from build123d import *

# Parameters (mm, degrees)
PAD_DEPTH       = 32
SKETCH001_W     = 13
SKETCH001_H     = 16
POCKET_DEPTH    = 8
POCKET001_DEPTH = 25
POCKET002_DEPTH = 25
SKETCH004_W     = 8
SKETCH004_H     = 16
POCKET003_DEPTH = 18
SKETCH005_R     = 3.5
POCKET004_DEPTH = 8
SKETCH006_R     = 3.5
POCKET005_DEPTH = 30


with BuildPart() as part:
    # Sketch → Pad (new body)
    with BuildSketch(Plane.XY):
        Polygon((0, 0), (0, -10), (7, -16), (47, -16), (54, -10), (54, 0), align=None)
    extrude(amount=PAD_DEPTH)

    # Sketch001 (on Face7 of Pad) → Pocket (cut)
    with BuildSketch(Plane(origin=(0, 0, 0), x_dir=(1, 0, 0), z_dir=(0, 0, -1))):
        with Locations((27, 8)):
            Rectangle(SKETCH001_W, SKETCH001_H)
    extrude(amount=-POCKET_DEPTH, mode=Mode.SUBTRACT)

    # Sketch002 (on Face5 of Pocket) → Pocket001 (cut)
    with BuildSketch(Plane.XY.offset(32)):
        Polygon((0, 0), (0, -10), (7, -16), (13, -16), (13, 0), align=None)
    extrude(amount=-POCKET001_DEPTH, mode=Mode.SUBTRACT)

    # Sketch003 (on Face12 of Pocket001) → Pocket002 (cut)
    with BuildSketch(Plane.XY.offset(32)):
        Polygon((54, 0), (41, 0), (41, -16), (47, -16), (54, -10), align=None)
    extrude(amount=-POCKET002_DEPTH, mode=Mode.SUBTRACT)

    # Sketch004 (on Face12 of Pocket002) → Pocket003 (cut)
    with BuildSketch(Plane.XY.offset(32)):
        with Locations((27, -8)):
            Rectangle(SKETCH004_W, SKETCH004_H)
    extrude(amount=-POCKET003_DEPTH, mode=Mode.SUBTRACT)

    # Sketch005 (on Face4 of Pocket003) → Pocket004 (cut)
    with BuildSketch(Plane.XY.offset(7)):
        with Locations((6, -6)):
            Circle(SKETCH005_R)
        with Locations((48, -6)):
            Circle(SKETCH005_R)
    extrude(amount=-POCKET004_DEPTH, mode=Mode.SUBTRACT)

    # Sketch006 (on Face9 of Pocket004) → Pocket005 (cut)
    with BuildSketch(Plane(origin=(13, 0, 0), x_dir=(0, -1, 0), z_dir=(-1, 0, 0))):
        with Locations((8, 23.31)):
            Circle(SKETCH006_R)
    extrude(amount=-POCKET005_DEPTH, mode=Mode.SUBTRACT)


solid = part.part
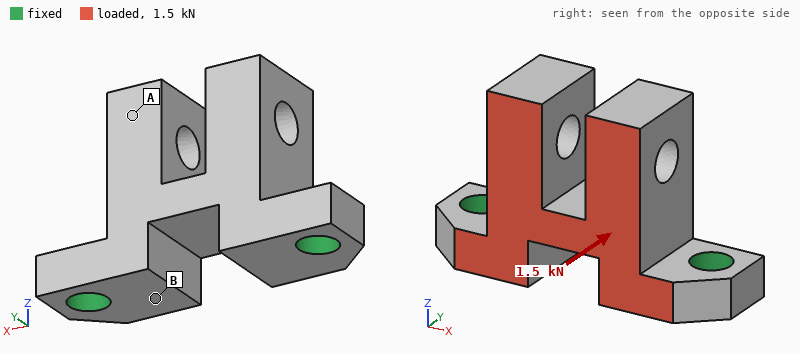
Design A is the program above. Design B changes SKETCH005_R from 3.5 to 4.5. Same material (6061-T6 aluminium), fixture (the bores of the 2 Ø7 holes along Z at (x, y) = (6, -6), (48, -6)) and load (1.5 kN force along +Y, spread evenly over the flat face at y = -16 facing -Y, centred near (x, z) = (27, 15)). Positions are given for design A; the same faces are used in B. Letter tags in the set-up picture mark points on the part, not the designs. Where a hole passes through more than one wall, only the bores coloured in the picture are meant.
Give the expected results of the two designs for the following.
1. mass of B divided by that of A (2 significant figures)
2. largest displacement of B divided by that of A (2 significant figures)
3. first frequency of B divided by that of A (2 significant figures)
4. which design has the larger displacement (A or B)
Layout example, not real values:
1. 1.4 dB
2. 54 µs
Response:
1. 0.97
2. 0.81
3. 1.1
4. A
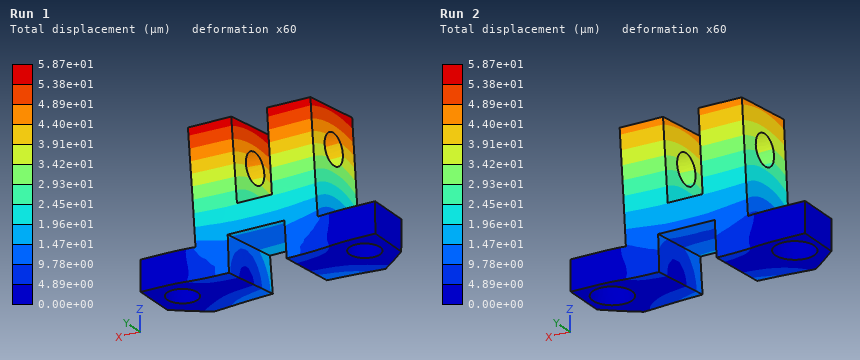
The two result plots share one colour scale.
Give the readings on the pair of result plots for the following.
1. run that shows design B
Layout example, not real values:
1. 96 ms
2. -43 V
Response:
1. Run 2
